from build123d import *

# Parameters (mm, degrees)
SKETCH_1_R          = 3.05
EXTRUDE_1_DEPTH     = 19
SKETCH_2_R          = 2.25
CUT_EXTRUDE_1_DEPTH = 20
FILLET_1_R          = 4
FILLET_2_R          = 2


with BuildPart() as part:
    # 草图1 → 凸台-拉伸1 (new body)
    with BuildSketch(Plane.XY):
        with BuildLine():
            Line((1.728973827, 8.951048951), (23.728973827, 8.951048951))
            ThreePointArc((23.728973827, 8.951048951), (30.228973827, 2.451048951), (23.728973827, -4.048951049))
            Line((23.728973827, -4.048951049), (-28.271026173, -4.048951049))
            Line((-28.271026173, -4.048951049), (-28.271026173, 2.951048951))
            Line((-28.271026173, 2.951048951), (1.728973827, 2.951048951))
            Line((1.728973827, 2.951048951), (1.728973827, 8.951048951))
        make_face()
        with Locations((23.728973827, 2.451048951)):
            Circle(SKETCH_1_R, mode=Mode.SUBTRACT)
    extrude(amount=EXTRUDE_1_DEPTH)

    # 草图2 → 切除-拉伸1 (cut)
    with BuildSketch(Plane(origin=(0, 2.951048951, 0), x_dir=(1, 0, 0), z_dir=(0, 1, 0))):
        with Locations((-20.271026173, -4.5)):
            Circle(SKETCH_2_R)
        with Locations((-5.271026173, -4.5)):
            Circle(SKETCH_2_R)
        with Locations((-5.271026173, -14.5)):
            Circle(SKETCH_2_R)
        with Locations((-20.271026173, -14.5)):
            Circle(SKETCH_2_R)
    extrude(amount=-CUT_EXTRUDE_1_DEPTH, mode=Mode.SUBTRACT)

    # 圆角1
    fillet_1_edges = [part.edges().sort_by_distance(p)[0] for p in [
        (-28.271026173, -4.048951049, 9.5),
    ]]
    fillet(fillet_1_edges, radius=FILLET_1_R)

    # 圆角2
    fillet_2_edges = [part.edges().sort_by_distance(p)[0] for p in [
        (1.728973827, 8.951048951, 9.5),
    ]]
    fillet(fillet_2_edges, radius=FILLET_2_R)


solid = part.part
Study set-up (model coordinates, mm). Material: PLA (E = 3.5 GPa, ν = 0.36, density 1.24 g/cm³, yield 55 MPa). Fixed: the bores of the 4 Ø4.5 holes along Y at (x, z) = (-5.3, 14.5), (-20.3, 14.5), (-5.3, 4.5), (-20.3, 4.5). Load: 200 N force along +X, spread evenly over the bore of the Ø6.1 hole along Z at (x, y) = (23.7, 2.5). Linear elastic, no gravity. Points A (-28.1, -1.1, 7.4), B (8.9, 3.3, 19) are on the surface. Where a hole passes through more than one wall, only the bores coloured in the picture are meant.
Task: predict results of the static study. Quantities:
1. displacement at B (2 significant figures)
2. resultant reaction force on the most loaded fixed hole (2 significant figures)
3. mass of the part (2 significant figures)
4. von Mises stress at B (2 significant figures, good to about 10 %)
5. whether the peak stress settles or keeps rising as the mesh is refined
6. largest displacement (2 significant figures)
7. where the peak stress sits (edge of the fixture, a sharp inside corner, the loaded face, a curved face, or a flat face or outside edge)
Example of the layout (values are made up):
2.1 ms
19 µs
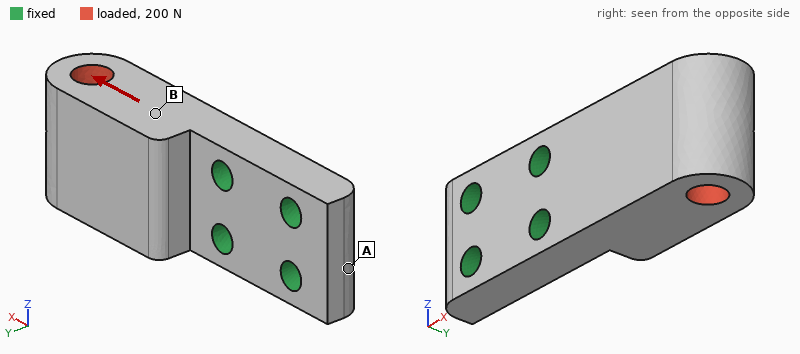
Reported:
27 µm
99 N
12 g
1.3 MPa
keeps rising
80 µm
edge of the fixture
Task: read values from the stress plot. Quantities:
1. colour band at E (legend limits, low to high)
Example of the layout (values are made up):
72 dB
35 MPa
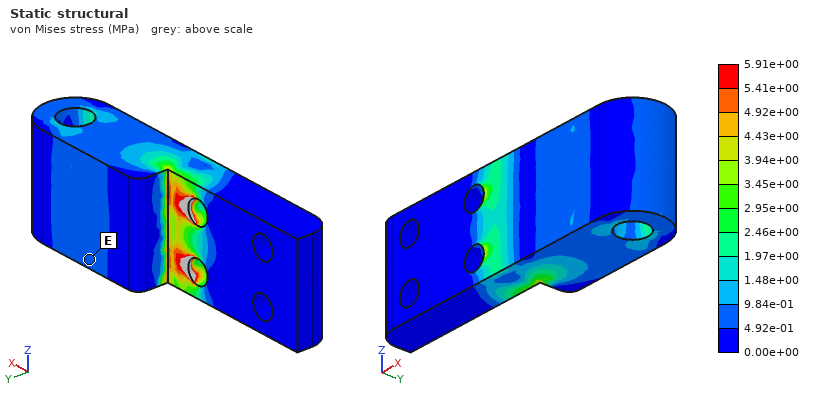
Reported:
4.92e-01 to 9.84e-01 MPa
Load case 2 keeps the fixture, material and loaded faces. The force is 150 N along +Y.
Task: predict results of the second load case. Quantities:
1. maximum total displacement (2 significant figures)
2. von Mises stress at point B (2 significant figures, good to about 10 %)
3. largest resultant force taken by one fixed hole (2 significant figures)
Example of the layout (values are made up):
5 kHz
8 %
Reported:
0.54 mm
3.4 MPa
84 N
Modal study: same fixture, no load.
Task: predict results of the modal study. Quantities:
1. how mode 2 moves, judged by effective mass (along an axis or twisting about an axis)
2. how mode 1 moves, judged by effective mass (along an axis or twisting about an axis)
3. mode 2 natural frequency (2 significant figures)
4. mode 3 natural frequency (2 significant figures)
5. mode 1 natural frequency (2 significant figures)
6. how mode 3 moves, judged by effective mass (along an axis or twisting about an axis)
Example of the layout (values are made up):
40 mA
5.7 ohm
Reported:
along Z
along Y
3200 Hz
5100 Hz
1500 Hz
twisting about X
